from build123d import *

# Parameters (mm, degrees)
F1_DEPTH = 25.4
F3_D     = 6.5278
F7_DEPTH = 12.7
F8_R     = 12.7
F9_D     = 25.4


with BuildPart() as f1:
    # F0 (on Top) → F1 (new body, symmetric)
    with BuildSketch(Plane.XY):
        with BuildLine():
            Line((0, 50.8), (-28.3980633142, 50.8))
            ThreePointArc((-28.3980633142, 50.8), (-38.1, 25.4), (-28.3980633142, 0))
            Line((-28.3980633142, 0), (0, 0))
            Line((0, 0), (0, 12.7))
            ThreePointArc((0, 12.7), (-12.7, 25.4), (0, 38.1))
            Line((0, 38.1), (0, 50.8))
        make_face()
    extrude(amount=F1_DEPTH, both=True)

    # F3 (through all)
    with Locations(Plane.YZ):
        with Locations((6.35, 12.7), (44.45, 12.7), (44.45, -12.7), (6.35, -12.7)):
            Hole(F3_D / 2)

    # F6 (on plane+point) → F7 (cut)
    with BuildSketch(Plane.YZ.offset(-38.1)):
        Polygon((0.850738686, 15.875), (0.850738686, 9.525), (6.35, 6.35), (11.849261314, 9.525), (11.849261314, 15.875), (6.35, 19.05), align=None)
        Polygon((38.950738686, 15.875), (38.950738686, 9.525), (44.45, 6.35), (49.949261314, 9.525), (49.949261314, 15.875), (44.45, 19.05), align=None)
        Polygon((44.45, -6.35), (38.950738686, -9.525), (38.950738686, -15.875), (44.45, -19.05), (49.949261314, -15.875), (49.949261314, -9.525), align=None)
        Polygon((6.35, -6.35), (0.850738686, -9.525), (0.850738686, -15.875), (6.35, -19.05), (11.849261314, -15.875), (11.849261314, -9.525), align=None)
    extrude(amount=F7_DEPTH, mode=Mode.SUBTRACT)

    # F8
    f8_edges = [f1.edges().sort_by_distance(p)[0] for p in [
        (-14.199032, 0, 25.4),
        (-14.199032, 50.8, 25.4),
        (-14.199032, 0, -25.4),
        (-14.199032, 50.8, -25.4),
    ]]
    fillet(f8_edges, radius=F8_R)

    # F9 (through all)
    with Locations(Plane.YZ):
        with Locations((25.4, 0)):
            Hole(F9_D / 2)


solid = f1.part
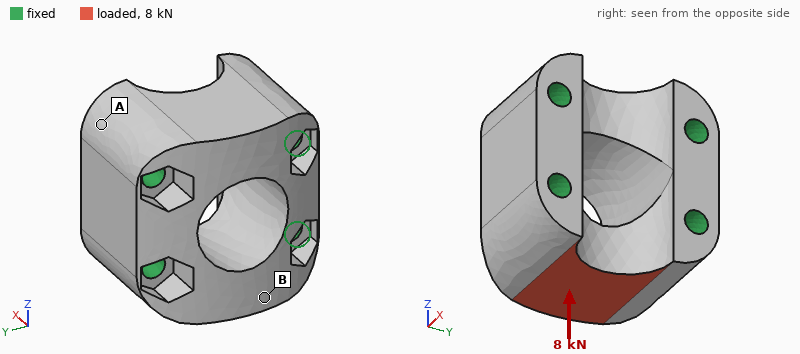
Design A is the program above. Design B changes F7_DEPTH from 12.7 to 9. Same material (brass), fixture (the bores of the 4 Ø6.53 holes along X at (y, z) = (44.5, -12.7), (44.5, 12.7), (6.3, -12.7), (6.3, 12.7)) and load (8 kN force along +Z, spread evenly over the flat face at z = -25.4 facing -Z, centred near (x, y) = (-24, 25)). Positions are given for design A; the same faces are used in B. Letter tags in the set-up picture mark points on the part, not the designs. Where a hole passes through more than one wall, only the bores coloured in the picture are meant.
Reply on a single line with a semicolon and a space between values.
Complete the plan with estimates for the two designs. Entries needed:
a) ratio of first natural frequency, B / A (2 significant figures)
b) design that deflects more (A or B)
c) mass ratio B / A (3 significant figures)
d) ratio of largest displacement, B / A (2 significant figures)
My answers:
1.2; A; 1.02; 0.82
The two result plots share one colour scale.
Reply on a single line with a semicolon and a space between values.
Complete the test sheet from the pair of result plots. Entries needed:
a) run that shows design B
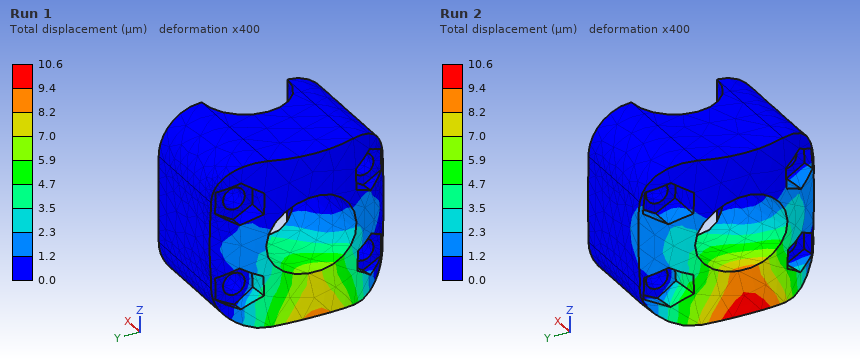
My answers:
Run 1
